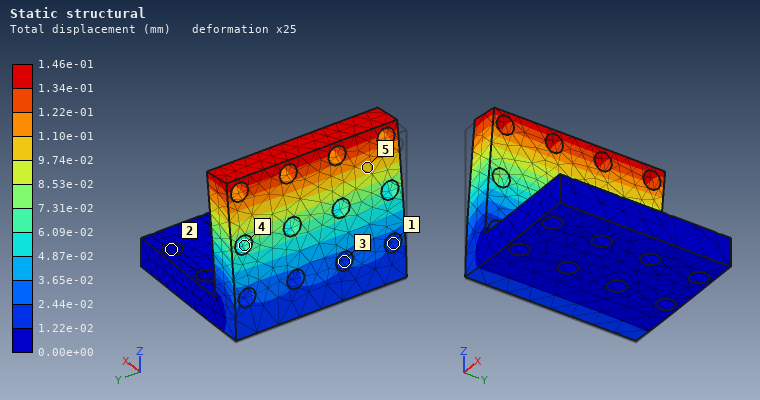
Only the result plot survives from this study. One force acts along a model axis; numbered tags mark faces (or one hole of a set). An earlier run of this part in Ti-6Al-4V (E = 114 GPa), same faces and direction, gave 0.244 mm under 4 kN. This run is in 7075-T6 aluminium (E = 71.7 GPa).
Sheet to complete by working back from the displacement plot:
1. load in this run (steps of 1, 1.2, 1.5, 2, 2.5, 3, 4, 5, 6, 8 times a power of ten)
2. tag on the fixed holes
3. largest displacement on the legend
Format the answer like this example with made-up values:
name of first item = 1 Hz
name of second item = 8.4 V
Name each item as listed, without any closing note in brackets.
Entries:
load in this run = 1.5 kN
tag on the fixed holes = 2
largest displacement on the legend = 1.46e-01 mm
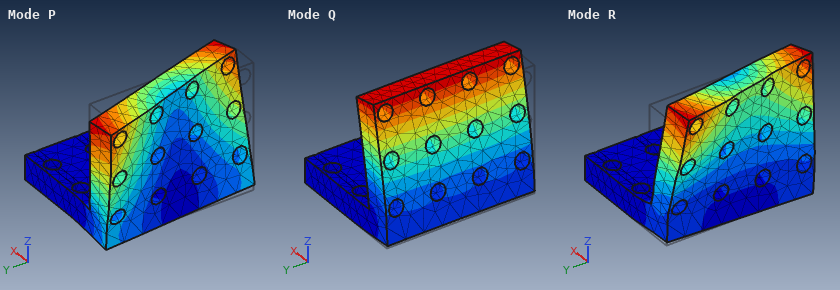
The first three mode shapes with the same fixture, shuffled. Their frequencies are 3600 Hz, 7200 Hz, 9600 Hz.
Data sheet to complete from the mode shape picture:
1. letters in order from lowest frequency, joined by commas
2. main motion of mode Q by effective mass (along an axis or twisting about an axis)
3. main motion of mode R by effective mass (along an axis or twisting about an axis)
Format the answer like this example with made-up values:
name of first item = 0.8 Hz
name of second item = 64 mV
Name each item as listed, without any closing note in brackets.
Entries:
letters in order from lowest frequency, joined by commas = Q, P, R
main motion of mode Q by effective mass = along X
main motion of mode R by effective mass = along Y
